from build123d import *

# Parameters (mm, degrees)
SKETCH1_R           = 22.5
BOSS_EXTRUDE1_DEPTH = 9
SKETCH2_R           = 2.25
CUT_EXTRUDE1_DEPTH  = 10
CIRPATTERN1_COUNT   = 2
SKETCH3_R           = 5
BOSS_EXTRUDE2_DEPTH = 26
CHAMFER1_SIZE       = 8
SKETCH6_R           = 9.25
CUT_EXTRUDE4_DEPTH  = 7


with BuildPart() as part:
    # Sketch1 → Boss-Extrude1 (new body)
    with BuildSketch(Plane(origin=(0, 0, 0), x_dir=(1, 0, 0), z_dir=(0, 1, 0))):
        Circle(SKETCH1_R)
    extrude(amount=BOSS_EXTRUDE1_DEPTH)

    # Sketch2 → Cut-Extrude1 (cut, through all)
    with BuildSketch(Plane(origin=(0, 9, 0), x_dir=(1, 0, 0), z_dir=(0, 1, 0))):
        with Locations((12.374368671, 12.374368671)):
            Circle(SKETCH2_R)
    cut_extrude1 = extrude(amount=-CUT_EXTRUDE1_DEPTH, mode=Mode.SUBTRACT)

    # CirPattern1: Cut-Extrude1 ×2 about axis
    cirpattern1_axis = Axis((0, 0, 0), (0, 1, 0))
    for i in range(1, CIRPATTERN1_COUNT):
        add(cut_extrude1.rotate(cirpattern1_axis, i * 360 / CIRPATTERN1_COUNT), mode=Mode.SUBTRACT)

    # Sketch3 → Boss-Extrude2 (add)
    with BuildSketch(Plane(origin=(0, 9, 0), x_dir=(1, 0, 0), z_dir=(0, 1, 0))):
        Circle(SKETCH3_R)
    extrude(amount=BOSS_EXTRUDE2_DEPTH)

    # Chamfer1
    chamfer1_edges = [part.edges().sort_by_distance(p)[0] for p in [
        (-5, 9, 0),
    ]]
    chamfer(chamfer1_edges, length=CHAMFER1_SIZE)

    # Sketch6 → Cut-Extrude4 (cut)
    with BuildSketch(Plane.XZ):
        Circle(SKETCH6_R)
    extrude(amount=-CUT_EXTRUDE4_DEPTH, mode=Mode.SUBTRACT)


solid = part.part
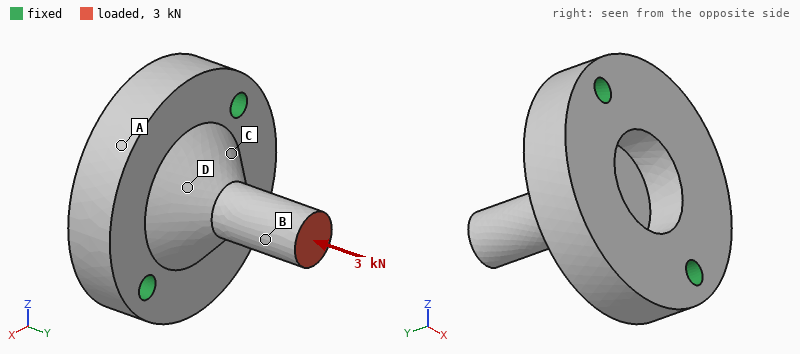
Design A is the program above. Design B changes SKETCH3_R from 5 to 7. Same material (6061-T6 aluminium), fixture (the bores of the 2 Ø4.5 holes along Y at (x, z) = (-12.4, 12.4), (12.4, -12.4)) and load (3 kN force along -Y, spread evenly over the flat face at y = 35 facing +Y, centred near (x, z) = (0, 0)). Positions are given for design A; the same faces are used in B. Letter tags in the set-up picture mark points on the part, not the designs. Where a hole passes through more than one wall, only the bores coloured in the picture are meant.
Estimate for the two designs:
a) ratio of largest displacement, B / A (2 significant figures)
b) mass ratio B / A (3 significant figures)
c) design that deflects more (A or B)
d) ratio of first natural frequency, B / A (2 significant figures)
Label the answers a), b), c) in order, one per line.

a) 0.62
b) 1.15
c) A
d) 0.92
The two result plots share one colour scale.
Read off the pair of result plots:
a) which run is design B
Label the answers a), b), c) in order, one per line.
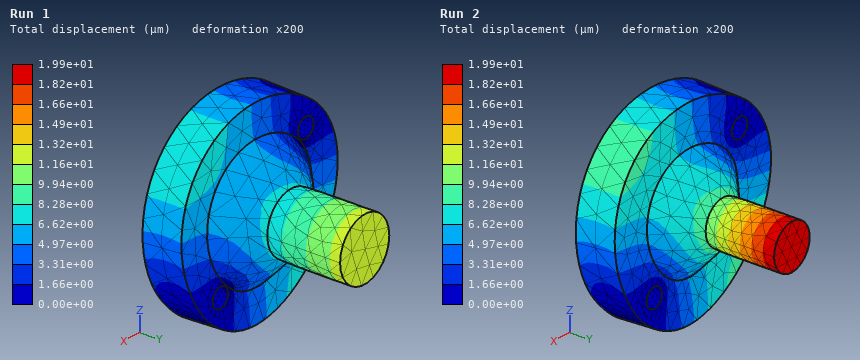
a) Run 1
